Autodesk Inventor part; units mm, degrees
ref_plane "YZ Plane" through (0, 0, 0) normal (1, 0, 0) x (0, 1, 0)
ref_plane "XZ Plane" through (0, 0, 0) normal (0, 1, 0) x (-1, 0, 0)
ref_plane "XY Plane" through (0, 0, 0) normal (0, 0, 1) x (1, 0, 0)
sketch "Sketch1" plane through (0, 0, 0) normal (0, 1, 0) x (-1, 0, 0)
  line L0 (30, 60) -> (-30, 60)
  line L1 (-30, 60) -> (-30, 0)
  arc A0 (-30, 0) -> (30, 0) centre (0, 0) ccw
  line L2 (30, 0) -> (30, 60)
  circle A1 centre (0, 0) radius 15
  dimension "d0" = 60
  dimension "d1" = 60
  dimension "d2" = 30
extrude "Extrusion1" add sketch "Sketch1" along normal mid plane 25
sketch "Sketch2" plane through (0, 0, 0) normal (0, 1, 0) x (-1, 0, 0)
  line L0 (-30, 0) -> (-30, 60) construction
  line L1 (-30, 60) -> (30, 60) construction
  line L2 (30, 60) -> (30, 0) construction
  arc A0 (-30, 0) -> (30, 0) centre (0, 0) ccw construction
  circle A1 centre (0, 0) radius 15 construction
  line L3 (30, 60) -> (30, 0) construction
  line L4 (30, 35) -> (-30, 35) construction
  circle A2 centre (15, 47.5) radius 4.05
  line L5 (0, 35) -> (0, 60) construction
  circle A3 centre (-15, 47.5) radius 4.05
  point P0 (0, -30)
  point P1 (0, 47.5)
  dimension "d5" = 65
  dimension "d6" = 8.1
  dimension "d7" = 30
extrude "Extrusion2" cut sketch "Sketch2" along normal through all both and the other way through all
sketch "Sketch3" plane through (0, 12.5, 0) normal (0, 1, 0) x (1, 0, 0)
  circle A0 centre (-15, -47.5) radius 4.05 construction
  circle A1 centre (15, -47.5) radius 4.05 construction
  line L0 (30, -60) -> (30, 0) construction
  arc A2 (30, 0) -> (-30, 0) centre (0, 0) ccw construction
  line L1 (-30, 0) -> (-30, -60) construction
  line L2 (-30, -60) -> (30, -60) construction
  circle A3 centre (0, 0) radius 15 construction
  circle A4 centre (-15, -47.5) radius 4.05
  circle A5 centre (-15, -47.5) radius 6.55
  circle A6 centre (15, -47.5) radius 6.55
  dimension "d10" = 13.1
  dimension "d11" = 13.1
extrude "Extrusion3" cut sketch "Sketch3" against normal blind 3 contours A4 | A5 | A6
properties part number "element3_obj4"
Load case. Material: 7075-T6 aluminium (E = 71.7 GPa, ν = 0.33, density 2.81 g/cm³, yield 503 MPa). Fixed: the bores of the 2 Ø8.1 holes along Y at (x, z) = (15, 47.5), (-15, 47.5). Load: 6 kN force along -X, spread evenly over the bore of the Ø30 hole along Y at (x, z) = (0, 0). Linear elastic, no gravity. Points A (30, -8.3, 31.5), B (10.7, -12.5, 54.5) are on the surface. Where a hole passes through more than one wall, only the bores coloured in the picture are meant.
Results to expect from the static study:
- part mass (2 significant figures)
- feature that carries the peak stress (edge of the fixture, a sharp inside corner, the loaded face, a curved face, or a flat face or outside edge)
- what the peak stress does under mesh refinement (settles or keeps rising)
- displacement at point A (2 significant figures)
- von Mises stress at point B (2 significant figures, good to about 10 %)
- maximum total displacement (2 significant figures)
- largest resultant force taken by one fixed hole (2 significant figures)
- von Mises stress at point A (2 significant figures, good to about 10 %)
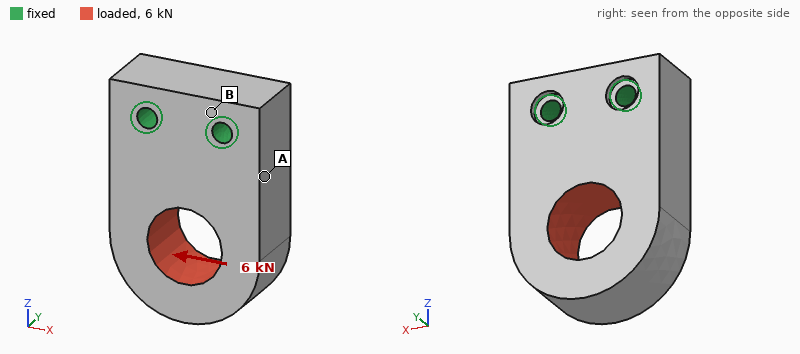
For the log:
290 g
edge of the fixture
keeps rising
9.4 µm
6.6 MPa
40 µm
8.3 kN
13 MPa
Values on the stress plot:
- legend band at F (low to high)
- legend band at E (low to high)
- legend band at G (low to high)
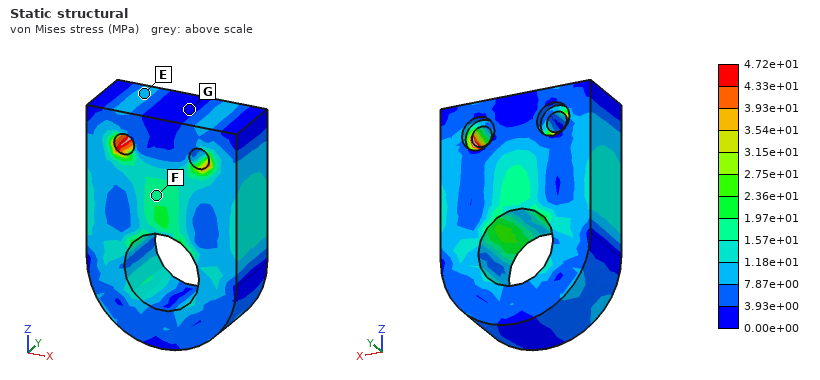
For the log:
1.57e+01 to 1.97e+01 MPa
7.87e+00 to 1.18e+01 MPa
0.00e+00 to 3.93e+00 MPa
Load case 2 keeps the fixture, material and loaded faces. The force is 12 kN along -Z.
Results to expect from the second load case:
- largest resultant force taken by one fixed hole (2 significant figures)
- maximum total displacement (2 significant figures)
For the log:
6.0 kN
14 µm
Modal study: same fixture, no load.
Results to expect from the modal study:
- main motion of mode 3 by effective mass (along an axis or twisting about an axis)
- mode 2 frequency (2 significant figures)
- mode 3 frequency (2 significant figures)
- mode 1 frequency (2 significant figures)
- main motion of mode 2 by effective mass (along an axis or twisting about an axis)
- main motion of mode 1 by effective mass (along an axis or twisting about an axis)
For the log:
twisting about Z
5600 Hz
7700 Hz
3500 Hz
along X
along Y
